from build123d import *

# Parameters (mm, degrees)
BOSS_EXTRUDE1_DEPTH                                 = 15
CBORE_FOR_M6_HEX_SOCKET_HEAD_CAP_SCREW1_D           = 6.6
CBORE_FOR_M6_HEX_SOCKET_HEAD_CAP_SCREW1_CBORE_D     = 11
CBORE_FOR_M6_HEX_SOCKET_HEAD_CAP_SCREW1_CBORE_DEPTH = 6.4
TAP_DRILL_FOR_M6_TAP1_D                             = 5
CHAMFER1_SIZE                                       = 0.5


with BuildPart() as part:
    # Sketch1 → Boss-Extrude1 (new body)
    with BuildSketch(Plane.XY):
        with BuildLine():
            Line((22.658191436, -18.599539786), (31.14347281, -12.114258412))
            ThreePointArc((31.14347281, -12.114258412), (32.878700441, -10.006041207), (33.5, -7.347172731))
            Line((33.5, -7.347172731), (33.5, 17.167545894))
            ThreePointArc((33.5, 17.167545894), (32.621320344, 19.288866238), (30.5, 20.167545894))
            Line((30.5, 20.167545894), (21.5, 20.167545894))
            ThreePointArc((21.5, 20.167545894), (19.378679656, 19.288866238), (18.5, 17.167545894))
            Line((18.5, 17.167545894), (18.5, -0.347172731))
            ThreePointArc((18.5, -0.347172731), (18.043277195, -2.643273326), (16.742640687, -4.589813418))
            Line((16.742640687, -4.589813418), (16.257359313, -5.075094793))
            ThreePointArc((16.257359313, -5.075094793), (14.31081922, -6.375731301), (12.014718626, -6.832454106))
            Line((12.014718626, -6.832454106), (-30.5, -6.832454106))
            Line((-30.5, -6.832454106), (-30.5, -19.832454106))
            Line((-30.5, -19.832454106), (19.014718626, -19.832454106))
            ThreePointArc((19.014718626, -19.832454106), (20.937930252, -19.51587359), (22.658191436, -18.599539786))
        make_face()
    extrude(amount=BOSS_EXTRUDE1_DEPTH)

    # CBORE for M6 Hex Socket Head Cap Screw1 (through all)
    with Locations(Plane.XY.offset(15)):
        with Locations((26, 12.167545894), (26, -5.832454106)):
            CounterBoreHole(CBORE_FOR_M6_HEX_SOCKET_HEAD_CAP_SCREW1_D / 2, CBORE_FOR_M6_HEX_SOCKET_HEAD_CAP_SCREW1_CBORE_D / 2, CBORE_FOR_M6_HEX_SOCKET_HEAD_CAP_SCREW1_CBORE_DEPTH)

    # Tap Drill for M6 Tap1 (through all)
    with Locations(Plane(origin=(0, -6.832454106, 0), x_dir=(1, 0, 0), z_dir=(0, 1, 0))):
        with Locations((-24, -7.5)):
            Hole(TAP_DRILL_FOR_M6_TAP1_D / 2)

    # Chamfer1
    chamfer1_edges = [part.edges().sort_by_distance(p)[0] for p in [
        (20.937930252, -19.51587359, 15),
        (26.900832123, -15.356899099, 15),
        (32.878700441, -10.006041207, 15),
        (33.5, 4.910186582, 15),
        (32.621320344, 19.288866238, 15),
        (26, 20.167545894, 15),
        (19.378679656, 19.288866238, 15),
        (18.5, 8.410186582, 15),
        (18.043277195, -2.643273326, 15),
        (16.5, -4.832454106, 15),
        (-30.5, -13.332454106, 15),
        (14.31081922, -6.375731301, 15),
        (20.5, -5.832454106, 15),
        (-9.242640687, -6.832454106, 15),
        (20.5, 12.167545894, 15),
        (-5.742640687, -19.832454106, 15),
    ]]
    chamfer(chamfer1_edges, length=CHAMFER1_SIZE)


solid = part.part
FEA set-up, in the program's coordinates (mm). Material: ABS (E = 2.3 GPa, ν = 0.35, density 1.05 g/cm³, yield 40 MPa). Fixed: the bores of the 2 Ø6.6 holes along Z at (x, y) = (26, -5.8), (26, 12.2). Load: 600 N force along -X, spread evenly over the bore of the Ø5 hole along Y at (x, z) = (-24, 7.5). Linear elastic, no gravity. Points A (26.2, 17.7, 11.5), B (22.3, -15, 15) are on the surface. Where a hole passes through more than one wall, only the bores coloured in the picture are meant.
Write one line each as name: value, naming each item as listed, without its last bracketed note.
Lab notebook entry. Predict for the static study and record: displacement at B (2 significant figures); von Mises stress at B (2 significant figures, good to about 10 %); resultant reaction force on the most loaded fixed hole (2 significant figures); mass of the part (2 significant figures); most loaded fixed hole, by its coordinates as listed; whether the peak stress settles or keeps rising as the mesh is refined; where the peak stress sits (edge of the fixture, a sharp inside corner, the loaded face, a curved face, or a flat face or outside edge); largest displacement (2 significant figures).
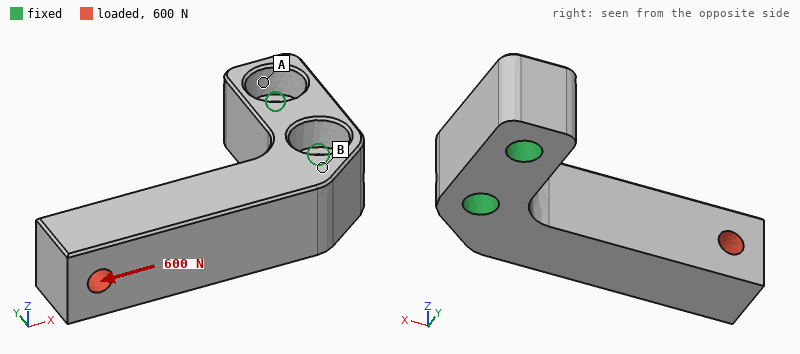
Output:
displacement at B: 0.089 mm
von Mises stress at B: 4.6 MPa
resultant reaction force on the most loaded fixed hole: 680 N
mass of the part: 16 g
most loaded fixed hole, by its coordinates as listed: (26, -5.8)
whether the peak stress settles or keeps rising as the mesh is refined: keeps rising
where the peak stress sits: edge of the fixture
largest displacement: 0.39 mm
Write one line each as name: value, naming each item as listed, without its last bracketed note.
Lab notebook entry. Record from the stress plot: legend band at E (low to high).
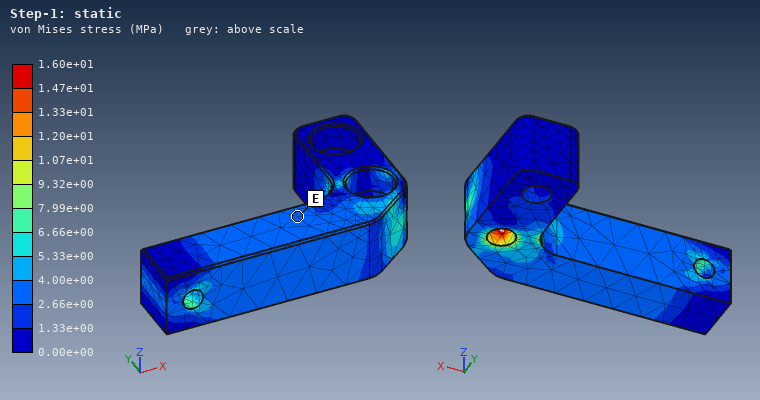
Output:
legend band at E: 2.66e+00 to 4.00e+00 MPa
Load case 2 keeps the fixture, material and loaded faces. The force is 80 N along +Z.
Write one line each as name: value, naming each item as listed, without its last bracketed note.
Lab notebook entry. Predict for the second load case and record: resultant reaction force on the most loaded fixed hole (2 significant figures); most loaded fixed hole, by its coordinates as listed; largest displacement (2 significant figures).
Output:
resultant reaction force on the most loaded fixed hole: 110 N
most loaded fixed hole, by its coordinates as listed: (26, -5.8)
largest displacement: 0.79 mm
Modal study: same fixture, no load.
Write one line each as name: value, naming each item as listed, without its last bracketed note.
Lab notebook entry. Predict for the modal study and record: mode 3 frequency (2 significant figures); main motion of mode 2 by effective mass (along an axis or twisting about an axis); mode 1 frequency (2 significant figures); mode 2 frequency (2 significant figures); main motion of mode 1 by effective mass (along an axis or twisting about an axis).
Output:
mode 3 frequency: 3500 Hz
main motion of mode 2 by effective mass: along Y
mode 1 frequency: 860 Hz
mode 2 frequency: 920 Hz
main motion of mode 1 by effective mass: along Z
